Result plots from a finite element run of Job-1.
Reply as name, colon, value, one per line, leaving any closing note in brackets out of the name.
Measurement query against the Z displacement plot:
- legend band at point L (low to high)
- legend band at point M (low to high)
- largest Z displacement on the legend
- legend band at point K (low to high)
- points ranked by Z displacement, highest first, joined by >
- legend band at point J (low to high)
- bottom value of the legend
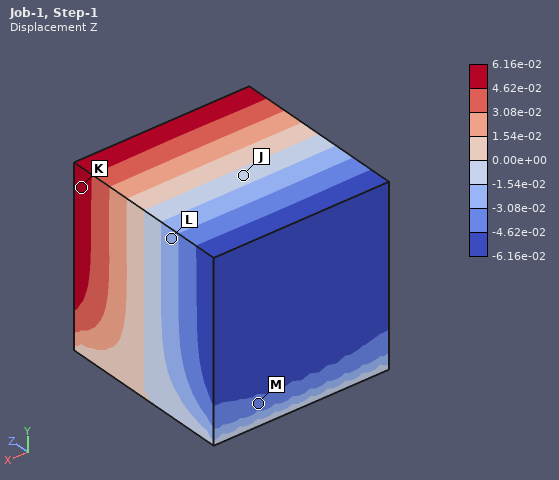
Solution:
legend band at point L: -3.08e-02 to -1.54e-02
legend band at point M: -4.62e-02 to -3.08e-02
largest Z displacement on the legend: 6.16e-02
legend band at point K: 4.62e-02 to 6.16e-02
points ranked by Z displacement, highest first, joined by >: K > J > L > M
legend band at point J: -1.54e-02 to 0.00e+00
bottom value of the legend: -6.16e-02
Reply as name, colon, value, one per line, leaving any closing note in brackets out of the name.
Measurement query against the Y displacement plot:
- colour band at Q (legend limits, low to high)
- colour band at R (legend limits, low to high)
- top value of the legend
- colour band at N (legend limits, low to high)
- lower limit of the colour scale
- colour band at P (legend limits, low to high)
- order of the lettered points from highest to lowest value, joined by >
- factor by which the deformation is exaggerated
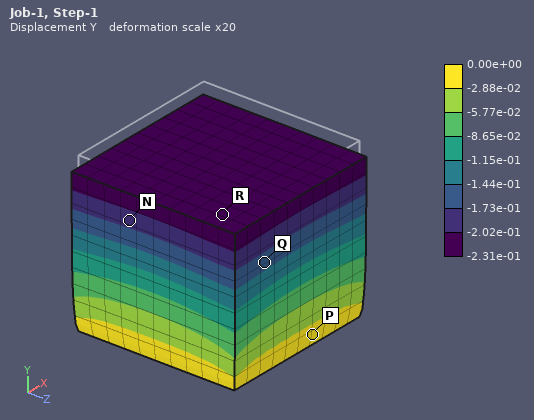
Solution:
colour band at Q: -1.73e-01 to -1.44e-01
colour band at R: -2.31e-01 to -2.02e-01
top value of the legend: 0.00e+00
colour band at N: -2.02e-01 to -1.73e-01
lower limit of the colour scale: -2.31e-01
colour band at P: -2.88e-02 to 0.00e+00
order of the lettered points from highest to lowest value, joined by >: P > Q > N > R
factor by which the deformation is exaggerated: 20
